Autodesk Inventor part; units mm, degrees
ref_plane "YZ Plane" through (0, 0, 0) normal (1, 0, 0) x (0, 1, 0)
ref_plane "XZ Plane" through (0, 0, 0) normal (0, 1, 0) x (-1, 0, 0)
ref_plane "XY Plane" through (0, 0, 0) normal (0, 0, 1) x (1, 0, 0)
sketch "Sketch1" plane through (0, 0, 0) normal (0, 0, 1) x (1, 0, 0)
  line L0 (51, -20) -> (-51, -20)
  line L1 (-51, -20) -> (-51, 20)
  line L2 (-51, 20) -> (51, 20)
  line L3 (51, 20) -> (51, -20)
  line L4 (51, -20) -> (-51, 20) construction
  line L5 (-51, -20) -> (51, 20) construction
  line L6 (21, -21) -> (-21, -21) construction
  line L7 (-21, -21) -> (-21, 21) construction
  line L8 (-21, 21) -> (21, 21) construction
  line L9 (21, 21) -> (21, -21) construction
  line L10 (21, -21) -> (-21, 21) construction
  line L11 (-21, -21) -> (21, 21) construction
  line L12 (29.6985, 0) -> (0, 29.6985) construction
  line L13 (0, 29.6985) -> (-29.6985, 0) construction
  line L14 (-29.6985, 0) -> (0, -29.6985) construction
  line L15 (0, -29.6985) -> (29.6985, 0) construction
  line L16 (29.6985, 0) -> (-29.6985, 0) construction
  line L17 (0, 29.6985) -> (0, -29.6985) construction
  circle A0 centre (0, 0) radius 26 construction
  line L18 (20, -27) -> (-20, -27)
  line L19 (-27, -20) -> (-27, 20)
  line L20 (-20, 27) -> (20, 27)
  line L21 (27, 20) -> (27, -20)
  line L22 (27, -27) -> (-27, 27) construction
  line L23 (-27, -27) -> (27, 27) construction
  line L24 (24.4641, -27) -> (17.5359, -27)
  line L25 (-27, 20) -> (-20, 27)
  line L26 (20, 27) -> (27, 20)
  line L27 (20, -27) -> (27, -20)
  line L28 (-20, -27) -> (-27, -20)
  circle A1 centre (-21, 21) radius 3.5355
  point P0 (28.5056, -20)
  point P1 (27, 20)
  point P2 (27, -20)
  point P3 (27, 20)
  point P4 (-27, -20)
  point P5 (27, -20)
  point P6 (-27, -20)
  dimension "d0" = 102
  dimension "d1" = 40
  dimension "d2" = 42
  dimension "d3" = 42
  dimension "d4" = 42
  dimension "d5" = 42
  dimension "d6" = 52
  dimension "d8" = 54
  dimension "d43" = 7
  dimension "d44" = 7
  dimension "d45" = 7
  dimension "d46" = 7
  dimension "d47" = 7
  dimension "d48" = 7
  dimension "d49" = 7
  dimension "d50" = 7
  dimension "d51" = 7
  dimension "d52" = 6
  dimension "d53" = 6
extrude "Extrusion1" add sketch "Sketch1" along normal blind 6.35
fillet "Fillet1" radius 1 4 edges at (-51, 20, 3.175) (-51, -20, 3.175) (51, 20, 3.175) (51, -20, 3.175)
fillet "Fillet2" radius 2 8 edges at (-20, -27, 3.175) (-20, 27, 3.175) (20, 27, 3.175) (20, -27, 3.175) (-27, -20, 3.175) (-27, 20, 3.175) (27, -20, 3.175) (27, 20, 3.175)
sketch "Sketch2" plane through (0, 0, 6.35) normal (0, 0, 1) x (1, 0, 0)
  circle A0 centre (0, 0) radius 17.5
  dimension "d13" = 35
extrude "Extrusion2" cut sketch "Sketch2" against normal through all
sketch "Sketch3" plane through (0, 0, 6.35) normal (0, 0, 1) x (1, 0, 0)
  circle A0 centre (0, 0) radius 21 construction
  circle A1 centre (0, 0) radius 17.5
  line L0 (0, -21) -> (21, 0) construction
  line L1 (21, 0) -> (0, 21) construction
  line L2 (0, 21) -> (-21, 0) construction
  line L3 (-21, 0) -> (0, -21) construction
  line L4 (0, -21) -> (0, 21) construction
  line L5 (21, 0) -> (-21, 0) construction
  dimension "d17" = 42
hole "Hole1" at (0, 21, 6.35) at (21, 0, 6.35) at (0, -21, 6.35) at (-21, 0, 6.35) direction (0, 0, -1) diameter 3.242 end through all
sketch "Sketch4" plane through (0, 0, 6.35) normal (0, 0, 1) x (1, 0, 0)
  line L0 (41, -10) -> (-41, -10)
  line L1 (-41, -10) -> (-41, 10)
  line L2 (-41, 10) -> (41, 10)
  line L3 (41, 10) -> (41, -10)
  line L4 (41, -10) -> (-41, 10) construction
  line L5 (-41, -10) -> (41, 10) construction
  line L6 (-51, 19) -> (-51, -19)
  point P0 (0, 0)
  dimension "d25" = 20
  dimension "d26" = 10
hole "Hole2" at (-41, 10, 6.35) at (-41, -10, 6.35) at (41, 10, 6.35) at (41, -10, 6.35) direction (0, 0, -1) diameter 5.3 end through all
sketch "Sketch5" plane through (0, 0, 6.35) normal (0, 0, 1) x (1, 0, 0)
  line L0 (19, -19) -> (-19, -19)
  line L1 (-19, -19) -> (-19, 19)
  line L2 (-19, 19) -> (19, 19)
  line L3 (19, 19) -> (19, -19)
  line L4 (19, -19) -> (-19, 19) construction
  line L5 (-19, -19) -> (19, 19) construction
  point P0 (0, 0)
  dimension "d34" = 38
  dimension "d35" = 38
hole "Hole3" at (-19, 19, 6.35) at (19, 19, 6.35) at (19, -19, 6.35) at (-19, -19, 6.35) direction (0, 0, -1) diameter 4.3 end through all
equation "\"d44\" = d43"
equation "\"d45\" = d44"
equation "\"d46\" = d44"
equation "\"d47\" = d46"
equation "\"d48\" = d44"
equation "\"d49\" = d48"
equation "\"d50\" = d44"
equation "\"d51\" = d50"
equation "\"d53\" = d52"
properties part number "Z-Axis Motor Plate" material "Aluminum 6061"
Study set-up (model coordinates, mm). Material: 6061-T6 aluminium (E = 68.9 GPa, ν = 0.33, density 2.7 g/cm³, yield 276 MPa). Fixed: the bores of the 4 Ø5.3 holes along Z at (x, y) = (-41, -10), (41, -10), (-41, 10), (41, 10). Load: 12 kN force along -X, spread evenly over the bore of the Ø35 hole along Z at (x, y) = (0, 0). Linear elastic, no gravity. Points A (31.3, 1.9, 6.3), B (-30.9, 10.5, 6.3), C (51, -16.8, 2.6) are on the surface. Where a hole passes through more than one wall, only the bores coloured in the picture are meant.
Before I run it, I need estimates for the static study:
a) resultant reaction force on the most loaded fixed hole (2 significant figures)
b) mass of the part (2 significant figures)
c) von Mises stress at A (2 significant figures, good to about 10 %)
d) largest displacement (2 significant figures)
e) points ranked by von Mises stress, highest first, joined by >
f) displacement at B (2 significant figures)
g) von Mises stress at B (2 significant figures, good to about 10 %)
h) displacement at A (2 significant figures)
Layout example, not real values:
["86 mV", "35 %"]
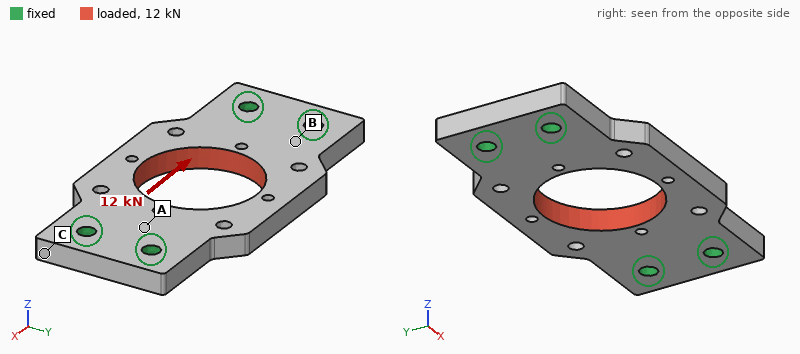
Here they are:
["3.0 kN", "62 g", "15 MPa", "18 µm", "B > A > C", "4.0 µm", "29 MPa", "3.3 µm"]
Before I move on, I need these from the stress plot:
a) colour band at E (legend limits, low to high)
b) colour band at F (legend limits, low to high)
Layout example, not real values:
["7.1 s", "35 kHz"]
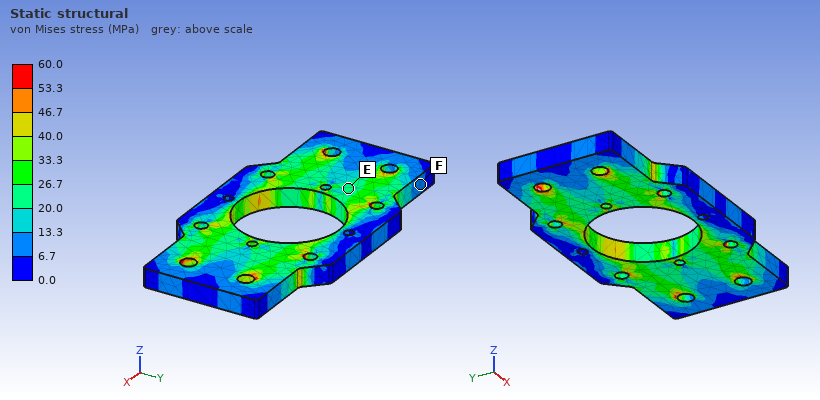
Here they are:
["20.0 to 26.7 MPa", "6.7 to 13.3 MPa"]
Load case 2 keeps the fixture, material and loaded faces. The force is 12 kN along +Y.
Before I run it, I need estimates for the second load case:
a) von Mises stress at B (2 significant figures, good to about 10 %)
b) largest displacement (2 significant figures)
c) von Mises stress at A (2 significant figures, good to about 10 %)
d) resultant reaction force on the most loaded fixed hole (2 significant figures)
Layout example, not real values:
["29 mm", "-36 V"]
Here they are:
["40 MPa", "53 µm", "67 MPa", "3.9 kN"]
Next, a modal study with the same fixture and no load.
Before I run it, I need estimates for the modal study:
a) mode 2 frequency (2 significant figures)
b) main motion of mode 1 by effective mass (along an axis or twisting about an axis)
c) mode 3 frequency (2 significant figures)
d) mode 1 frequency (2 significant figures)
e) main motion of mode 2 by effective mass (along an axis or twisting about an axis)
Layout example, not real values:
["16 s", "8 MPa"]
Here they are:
["5200 Hz", "along Z", "11 kHz", "4900 Hz", "twisting about X"]
